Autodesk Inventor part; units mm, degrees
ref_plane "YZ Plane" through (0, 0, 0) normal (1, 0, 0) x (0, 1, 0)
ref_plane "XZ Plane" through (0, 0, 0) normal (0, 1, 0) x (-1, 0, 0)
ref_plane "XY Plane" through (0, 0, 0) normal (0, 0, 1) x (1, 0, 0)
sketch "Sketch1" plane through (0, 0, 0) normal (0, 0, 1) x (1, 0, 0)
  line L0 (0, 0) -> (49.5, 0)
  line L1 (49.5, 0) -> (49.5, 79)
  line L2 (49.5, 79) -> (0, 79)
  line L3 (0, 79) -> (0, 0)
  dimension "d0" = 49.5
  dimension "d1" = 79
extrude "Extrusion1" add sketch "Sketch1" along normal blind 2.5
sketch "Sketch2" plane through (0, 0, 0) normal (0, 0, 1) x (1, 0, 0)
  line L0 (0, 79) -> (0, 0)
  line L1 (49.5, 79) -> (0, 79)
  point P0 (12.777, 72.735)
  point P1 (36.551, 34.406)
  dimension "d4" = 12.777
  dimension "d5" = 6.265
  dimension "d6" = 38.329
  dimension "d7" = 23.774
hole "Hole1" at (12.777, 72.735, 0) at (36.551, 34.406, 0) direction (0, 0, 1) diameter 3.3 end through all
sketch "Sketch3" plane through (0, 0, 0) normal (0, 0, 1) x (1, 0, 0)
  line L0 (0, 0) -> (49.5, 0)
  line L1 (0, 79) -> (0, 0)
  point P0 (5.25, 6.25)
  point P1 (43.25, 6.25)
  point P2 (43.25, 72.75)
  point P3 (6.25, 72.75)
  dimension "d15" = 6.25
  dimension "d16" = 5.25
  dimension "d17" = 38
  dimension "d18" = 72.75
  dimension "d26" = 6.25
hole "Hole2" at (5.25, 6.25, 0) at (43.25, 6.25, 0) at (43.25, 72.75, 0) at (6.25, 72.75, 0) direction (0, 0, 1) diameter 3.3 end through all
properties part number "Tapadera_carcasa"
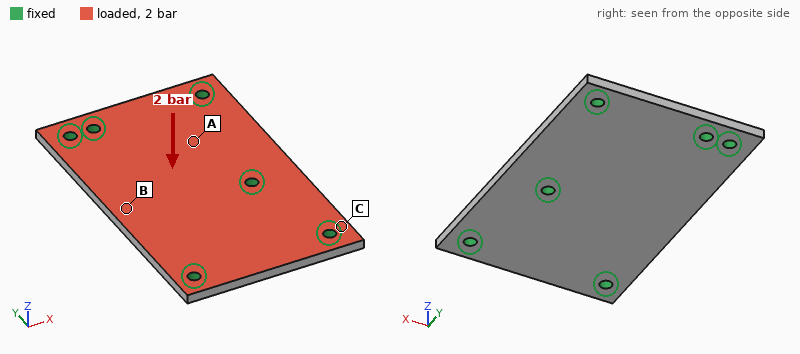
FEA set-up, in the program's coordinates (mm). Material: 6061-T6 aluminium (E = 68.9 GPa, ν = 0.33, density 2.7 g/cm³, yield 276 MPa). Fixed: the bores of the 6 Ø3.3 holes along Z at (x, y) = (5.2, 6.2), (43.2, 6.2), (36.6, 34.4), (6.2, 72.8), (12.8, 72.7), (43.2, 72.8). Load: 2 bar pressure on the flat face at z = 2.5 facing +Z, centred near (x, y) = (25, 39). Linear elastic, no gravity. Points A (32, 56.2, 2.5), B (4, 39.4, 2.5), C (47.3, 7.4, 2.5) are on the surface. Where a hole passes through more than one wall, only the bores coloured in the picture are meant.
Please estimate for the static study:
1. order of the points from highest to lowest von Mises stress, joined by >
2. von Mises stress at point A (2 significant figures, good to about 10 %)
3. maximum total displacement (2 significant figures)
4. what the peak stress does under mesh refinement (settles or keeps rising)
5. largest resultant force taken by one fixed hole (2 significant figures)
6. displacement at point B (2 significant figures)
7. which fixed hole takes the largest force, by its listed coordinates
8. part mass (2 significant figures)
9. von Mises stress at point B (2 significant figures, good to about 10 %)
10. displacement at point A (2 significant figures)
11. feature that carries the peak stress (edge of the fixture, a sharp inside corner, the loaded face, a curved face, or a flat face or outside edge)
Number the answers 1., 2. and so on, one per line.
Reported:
1. B > A > C
2. 12 MPa
3. 91 µm
4. keeps rising
5. 260 N
6. 81 µm
7. (36.6, 34.4)
8. 26 g
9. 23 MPa
10. 20 µm
11. edge of the fixture
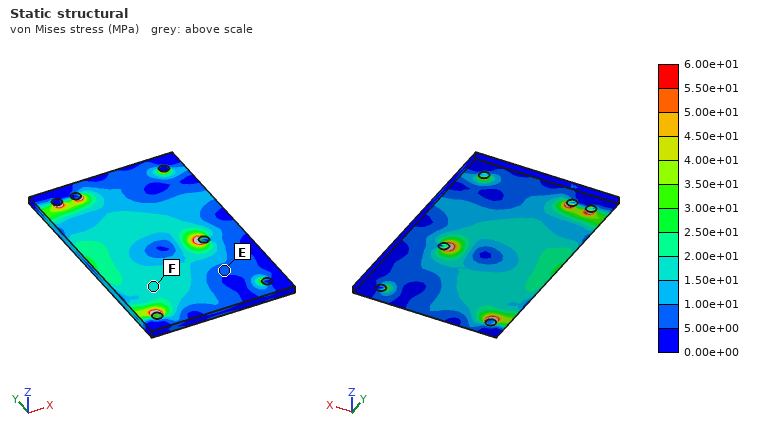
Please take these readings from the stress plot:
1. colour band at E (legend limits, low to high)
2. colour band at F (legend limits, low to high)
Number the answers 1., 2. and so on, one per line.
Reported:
1. 5.00e+00 to 1.00e+01 MPa
2. 1.50e+01 to 2.00e+01 MPa
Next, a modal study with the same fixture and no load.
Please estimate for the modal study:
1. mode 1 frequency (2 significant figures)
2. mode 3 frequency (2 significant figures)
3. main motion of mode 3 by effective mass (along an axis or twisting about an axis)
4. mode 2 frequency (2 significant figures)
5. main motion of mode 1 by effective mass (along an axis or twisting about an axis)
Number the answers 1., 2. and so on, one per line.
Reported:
1. 3800 Hz
2. 8500 Hz
3. along Z
4. 7700 Hz
5. along Z
